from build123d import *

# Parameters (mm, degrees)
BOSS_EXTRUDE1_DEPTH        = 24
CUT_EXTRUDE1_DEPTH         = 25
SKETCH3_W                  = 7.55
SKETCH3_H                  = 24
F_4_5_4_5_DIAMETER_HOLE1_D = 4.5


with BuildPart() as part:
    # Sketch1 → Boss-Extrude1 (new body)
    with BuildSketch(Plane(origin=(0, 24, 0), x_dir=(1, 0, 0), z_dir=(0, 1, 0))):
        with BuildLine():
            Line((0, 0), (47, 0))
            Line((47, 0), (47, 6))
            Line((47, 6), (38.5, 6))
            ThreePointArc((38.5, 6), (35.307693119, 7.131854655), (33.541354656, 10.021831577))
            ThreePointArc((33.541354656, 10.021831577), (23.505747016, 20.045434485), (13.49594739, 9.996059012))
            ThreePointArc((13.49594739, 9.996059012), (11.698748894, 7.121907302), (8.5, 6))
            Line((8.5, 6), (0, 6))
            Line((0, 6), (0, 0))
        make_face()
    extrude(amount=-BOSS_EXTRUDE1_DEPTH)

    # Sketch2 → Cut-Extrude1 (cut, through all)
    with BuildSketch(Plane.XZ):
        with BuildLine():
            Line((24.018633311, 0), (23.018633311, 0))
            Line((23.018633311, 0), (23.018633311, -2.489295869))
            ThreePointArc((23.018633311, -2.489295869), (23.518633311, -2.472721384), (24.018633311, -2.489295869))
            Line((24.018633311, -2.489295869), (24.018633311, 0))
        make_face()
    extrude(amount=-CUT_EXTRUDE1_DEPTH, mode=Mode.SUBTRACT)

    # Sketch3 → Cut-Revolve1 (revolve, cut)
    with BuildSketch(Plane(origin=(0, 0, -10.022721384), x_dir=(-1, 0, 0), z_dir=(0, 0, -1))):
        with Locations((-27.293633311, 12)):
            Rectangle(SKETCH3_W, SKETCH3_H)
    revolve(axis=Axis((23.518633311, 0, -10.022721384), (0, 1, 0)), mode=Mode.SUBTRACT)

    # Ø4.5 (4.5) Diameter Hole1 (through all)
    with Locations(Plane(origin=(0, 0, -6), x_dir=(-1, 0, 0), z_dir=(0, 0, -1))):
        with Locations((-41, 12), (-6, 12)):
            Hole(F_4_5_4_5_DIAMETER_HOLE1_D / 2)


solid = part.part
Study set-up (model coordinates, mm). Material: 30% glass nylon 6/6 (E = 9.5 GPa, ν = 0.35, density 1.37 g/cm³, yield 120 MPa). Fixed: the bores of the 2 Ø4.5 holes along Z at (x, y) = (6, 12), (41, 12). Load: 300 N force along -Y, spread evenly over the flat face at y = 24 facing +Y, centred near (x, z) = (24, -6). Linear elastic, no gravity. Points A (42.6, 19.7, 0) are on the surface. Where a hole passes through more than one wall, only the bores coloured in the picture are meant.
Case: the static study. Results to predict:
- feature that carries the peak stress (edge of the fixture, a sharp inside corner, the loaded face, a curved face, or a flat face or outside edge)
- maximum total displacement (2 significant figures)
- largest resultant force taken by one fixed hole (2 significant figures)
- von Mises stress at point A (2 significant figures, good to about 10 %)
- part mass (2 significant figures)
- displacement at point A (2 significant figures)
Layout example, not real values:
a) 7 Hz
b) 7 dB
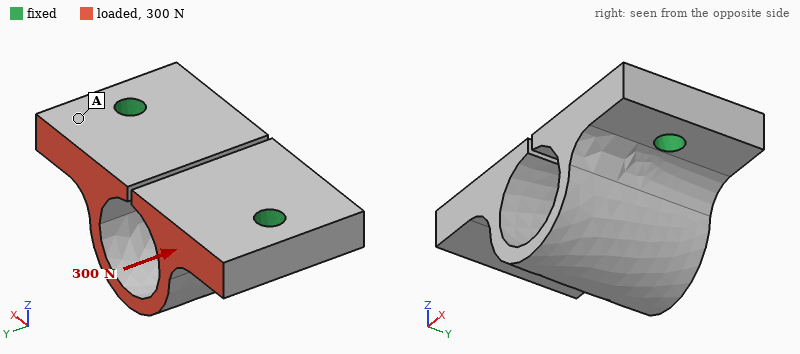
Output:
a) edge of the fixture
b) 25 µm
c) 150 N
d) 1.8 MPa
e) 11 g
f) 5.2 µm
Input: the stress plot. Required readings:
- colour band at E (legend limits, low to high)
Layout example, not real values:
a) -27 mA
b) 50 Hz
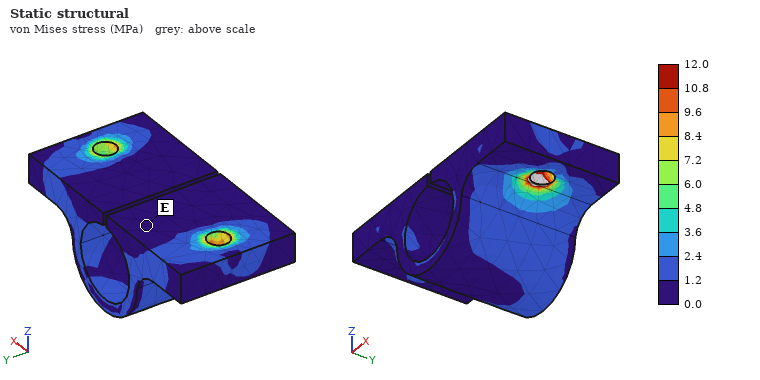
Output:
a) 0.0 to 1.2 MPa
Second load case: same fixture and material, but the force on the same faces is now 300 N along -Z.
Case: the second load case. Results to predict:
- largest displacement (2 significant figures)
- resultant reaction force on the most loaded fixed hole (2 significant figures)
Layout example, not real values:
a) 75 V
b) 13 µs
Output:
a) 52 µm
b) 150 N
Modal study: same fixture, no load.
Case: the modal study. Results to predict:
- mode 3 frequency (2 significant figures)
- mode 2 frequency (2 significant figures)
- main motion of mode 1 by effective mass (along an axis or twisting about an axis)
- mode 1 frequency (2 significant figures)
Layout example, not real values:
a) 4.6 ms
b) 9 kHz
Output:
a) 8400 Hz
b) 7500 Hz
c) along Y
d) 5900 Hz
